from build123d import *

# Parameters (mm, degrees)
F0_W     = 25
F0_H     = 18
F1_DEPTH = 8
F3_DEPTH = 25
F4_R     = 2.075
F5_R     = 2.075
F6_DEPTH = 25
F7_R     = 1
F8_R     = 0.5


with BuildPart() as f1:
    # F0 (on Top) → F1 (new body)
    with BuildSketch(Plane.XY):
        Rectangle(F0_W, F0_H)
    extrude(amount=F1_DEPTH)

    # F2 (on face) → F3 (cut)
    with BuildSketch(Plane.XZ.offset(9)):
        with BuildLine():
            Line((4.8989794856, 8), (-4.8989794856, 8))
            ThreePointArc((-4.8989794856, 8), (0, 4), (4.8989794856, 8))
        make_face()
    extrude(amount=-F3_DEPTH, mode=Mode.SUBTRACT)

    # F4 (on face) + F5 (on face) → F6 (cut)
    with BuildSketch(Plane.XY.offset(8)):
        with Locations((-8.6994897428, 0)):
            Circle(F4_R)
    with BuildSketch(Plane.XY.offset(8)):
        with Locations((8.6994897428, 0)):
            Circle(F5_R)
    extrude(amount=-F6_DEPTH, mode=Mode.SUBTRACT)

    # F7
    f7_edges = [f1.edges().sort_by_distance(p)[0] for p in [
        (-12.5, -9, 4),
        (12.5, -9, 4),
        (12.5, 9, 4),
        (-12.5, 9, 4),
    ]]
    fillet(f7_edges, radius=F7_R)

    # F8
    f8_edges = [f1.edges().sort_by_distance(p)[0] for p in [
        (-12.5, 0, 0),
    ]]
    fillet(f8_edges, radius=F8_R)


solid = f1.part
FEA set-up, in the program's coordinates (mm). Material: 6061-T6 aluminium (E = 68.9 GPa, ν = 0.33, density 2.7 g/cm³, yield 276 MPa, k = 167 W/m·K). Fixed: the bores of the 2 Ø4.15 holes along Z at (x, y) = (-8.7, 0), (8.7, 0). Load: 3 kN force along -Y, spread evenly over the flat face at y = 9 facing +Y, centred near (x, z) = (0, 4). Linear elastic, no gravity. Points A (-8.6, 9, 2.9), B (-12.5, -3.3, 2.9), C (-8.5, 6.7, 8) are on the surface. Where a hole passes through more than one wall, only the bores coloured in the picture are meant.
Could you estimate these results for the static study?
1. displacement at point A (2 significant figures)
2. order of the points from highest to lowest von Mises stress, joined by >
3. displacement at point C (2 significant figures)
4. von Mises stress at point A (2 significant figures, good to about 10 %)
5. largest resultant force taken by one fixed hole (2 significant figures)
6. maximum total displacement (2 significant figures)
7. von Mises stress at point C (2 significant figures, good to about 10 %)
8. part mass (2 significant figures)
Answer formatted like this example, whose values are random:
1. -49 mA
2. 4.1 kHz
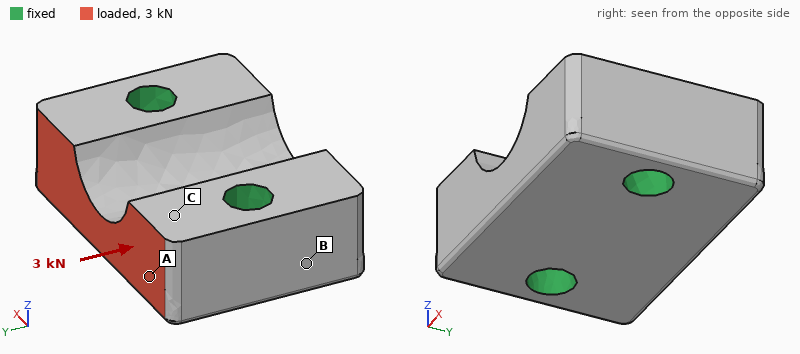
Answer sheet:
1. 2.3 µm
2. C > A > B
3. 1.9 µm
4. 16 MPa
5. 1.5 kN
6. 3.3 µm
7. 24 MPa
8. 7.7 g
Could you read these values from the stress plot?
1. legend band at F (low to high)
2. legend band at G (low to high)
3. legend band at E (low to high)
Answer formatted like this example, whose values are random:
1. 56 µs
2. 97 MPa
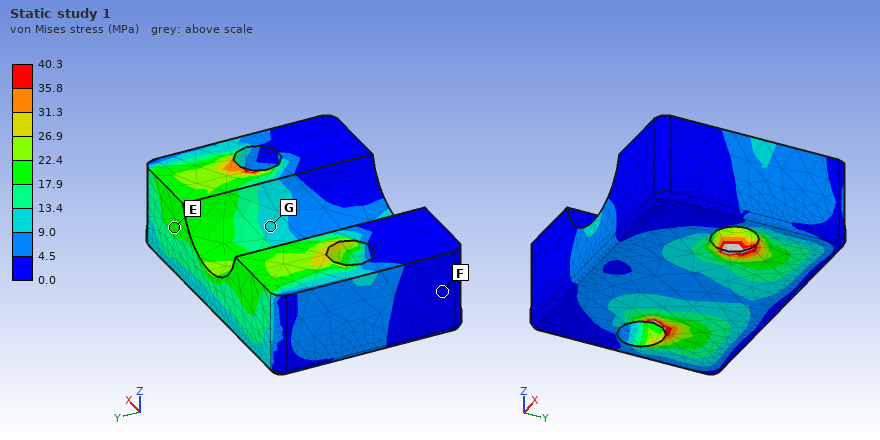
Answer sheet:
1. 0.0 to 4.5 MPa
2. 9.0 to 13.4 MPa
3. 17.9 to 22.4 MPa
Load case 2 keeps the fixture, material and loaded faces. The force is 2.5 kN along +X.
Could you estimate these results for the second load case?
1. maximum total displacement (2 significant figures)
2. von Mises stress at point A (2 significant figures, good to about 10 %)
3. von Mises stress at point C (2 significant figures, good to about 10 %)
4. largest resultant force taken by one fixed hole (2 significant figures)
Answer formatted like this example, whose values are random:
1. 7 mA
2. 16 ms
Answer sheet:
1. 10 µm
2. 36 MPa
3. 26 MPa
4. 1.5 kN
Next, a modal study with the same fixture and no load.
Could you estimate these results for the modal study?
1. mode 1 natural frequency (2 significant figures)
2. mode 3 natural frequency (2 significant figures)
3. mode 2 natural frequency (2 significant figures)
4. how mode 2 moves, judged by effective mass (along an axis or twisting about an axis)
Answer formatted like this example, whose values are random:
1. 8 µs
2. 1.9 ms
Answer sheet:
1. 55 kHz
2. 68 kHz
3. 61 kHz
4. along Z
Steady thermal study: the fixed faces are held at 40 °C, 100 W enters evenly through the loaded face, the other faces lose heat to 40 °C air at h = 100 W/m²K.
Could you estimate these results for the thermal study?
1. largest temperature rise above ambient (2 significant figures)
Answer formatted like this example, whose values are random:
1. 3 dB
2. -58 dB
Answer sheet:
1. 33 K
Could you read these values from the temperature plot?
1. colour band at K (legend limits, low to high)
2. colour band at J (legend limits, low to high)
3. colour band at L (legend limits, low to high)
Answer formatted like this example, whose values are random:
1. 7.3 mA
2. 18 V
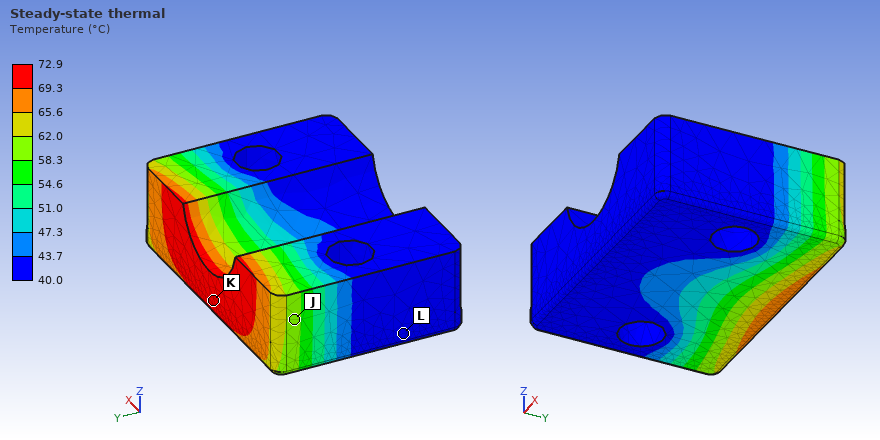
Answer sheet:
1. 69.3 to 72.9 °C
2. 58.3 to 62.0 °C
3. 40.0 to 43.7 °C
